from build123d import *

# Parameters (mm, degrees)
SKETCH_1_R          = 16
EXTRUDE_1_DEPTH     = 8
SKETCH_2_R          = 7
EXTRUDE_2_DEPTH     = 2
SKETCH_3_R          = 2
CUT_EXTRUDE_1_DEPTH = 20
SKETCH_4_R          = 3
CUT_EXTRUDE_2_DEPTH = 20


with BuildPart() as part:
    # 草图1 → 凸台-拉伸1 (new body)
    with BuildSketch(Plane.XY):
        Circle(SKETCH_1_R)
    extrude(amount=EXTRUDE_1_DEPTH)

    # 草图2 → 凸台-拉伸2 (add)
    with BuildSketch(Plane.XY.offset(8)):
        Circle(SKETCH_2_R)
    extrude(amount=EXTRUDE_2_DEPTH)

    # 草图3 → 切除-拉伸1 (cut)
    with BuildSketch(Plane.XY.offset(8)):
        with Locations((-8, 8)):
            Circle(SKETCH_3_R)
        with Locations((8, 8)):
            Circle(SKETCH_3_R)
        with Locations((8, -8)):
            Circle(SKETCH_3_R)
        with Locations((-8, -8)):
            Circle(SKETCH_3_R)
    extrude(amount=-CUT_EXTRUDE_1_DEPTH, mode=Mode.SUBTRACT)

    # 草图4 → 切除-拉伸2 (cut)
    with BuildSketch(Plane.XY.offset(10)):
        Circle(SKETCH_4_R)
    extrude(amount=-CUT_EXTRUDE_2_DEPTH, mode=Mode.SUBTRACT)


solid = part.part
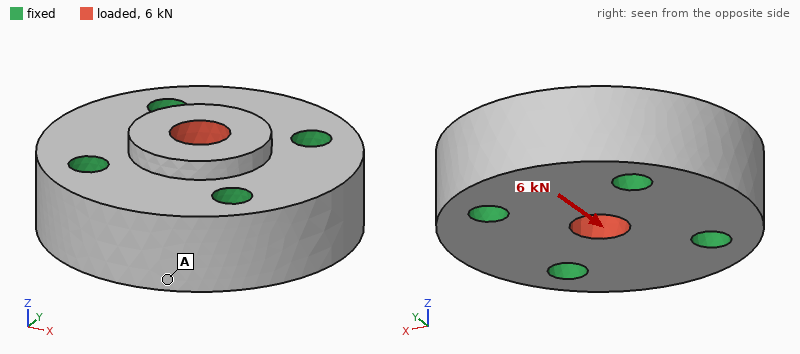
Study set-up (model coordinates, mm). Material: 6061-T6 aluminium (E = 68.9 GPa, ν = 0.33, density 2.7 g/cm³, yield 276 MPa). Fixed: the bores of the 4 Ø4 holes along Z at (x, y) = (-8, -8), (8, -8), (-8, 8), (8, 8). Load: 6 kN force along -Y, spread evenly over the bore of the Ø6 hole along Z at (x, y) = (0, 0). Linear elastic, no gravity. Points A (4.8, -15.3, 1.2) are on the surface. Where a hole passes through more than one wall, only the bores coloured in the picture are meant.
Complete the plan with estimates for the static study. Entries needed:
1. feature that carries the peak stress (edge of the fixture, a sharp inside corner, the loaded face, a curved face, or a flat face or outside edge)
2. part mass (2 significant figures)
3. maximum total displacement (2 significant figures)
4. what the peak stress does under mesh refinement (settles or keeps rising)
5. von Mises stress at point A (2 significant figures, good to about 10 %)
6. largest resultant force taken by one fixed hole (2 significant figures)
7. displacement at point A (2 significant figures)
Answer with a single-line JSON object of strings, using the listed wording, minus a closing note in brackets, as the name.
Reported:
{"feature that carries the peak stress": "edge of the fixture", "part mass": "16 g", "maximum total displacement": "5.8 µm", "what the peak stress does under mesh refinement": "keeps rising", "von Mises stress at point A": "7.7 MPa", "largest resultant force taken by one fixed hole": "1.6 kN", "displacement at point A": "1.1 µm"}
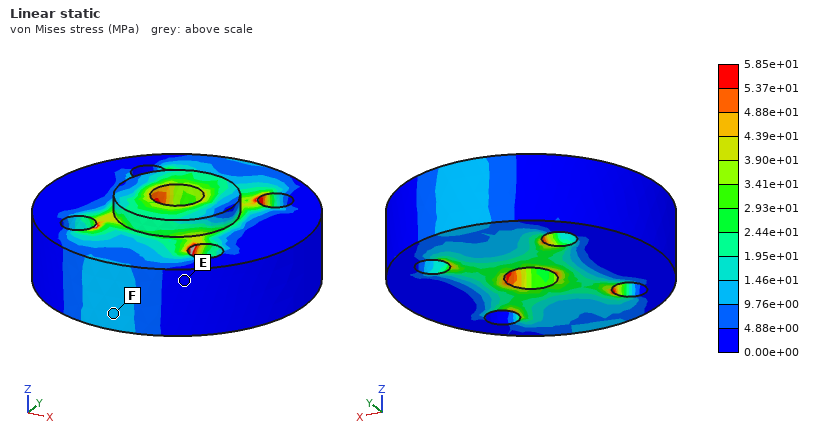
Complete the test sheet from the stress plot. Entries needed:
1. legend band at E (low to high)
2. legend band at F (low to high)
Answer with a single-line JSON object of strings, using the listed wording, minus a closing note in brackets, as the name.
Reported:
{"legend band at E": "0.00e+00 to 4.88e+00 MPa", "legend band at F": "9.76e+00 to 1.46e+01 MPa"}
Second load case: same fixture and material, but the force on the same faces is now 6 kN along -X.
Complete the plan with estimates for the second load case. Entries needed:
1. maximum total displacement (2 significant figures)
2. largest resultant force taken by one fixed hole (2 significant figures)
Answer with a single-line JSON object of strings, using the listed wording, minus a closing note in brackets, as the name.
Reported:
{"maximum total displacement": "5.8 µm", "largest resultant force taken by one fixed hole": "1.6 kN"}
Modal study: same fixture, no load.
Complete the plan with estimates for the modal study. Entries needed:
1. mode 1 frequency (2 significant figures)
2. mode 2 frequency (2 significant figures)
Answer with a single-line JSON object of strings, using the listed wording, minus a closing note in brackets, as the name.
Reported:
{"mode 1 frequency": "68 kHz", "mode 2 frequency": "69 kHz"}
